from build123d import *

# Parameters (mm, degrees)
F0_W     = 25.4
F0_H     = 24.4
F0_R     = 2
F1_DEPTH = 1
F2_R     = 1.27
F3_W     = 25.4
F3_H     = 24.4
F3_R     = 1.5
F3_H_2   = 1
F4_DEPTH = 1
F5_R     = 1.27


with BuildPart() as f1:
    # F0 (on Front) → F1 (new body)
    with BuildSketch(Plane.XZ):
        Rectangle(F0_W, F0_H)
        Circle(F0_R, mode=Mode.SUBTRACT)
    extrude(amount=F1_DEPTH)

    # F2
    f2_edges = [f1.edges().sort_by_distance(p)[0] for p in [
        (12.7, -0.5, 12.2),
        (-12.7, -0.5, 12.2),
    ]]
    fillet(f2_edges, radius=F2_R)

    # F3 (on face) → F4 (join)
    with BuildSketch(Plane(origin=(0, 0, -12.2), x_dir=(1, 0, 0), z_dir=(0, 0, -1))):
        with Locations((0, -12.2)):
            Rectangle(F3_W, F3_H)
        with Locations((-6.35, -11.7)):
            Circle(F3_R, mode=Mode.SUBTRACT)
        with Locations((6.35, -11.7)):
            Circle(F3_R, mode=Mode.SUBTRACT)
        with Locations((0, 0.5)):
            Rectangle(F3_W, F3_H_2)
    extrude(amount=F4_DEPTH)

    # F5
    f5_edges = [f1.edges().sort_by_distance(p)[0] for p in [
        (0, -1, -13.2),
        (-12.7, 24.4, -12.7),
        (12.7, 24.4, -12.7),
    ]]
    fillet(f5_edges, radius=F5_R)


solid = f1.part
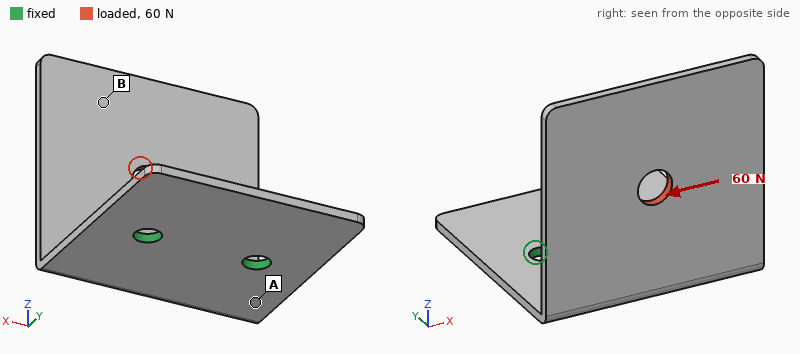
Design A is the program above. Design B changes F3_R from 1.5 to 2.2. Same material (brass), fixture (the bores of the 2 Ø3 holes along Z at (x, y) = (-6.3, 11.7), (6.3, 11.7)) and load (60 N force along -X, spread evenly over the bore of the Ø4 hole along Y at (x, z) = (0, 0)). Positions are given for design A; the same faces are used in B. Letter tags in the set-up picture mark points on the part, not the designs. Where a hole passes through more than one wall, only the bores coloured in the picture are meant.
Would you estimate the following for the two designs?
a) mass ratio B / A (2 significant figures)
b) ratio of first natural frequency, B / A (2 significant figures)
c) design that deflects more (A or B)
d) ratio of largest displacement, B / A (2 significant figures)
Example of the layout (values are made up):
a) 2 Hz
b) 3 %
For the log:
a) 0.99
b) 1.0
c) A
d) 0.86
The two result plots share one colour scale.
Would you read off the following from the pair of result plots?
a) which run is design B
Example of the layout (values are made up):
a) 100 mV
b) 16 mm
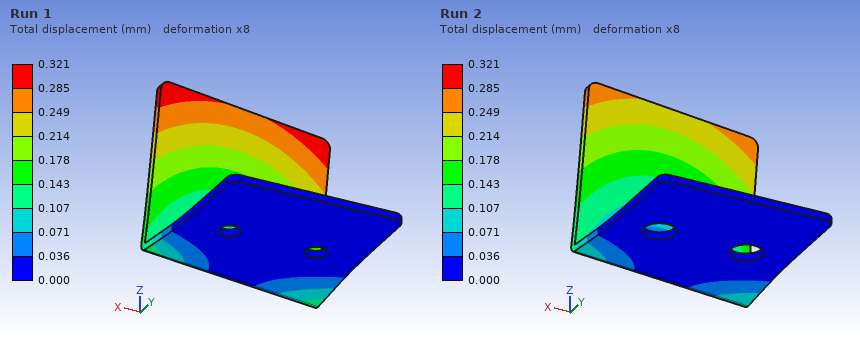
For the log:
a) Run 2
